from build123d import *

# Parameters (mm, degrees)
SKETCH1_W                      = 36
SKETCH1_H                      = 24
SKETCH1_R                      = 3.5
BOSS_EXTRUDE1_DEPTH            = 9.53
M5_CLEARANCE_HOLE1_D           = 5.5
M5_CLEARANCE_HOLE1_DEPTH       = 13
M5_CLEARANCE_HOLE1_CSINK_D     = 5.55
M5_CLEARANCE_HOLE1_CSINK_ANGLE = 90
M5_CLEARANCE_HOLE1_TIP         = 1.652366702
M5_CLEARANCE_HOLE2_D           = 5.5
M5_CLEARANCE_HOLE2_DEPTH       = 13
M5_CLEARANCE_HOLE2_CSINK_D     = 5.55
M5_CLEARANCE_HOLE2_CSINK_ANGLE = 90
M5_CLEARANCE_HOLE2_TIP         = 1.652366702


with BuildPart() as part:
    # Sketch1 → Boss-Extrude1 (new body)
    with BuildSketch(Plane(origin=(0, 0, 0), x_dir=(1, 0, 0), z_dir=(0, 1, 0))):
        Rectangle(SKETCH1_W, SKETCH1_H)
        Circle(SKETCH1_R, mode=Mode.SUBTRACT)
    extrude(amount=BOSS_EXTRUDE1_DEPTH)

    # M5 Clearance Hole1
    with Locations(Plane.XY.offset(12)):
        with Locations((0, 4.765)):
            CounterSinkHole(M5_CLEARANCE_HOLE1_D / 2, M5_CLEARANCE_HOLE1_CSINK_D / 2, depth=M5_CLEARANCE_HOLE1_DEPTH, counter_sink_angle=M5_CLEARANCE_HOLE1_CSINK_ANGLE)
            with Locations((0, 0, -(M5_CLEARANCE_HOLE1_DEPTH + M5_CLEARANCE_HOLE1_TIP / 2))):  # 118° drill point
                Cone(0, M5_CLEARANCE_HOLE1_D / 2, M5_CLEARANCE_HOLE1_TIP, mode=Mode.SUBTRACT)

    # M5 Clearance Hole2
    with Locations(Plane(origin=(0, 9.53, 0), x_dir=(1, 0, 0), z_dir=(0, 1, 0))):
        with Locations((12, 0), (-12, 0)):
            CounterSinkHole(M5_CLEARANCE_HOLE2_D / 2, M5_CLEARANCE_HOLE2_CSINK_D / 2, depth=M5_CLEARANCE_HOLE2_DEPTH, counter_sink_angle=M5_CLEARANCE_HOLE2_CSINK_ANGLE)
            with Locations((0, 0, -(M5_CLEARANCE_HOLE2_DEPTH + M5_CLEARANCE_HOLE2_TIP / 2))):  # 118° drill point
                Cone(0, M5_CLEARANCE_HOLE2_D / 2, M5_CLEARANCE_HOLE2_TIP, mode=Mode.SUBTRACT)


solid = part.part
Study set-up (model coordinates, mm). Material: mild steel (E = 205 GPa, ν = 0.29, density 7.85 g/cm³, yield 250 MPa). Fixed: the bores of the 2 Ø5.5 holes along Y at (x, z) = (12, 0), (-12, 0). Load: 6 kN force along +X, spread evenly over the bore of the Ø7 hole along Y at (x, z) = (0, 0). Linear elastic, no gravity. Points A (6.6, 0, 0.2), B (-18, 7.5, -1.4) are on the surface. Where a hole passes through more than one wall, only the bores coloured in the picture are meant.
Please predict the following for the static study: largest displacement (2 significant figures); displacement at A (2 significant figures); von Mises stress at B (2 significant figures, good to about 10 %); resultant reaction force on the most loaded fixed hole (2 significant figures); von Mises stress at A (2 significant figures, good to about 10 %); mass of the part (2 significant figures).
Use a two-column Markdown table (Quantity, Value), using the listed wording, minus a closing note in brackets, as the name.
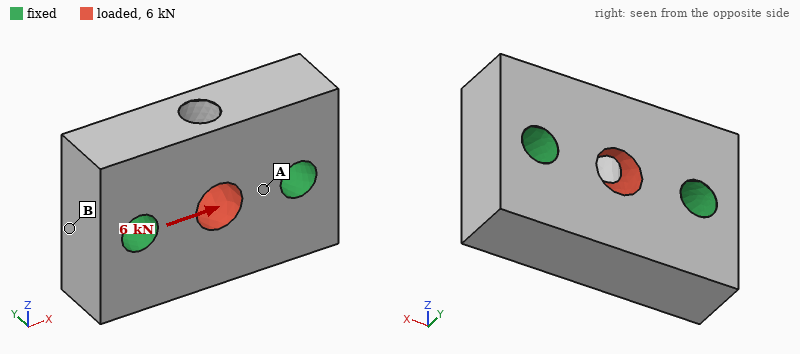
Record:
| Quantity | Value |
|---|---|
| largest displacement | 1.6 µm |
| displacement at A | 0.55 µm |
| von Mises stress at B | 10.0 MPa |
| resultant reaction force on the most loaded fixed hole | 3.0 kN |
| von Mises stress at A | 40 MPa |
| mass of the part | 57 g |
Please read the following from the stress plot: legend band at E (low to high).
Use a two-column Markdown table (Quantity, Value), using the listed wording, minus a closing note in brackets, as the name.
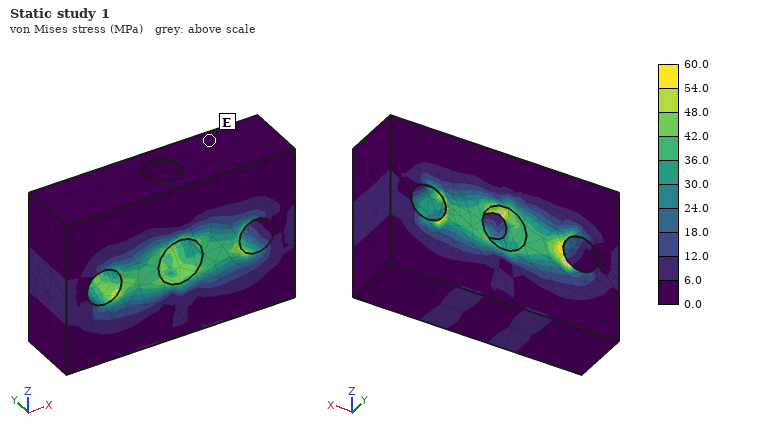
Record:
| Quantity | Value |
|---|---|
| legend band at E | 0.0 to 6.0 MPa |
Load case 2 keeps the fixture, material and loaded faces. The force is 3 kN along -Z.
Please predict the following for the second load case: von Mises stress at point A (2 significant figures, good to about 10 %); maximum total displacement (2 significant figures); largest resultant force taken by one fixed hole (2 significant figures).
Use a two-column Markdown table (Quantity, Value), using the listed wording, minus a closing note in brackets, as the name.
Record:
| Quantity | Value |
|---|---|
| von Mises stress at point A | 17 MPa |
| maximum total displacement | 1.4 µm |
| largest resultant force taken by one fixed hole | 1.5 kN |
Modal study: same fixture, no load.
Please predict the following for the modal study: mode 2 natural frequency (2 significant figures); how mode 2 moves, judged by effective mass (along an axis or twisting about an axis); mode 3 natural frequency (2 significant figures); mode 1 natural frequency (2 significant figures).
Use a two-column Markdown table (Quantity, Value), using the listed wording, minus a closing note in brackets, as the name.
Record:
| Quantity | Value |
|---|---|
| mode 2 natural frequency | 41 kHz |
| how mode 2 moves, judged by effective mass | along Y |
| mode 3 natural frequency | 50 kHz |
| mode 1 natural frequency | 36 kHz |
